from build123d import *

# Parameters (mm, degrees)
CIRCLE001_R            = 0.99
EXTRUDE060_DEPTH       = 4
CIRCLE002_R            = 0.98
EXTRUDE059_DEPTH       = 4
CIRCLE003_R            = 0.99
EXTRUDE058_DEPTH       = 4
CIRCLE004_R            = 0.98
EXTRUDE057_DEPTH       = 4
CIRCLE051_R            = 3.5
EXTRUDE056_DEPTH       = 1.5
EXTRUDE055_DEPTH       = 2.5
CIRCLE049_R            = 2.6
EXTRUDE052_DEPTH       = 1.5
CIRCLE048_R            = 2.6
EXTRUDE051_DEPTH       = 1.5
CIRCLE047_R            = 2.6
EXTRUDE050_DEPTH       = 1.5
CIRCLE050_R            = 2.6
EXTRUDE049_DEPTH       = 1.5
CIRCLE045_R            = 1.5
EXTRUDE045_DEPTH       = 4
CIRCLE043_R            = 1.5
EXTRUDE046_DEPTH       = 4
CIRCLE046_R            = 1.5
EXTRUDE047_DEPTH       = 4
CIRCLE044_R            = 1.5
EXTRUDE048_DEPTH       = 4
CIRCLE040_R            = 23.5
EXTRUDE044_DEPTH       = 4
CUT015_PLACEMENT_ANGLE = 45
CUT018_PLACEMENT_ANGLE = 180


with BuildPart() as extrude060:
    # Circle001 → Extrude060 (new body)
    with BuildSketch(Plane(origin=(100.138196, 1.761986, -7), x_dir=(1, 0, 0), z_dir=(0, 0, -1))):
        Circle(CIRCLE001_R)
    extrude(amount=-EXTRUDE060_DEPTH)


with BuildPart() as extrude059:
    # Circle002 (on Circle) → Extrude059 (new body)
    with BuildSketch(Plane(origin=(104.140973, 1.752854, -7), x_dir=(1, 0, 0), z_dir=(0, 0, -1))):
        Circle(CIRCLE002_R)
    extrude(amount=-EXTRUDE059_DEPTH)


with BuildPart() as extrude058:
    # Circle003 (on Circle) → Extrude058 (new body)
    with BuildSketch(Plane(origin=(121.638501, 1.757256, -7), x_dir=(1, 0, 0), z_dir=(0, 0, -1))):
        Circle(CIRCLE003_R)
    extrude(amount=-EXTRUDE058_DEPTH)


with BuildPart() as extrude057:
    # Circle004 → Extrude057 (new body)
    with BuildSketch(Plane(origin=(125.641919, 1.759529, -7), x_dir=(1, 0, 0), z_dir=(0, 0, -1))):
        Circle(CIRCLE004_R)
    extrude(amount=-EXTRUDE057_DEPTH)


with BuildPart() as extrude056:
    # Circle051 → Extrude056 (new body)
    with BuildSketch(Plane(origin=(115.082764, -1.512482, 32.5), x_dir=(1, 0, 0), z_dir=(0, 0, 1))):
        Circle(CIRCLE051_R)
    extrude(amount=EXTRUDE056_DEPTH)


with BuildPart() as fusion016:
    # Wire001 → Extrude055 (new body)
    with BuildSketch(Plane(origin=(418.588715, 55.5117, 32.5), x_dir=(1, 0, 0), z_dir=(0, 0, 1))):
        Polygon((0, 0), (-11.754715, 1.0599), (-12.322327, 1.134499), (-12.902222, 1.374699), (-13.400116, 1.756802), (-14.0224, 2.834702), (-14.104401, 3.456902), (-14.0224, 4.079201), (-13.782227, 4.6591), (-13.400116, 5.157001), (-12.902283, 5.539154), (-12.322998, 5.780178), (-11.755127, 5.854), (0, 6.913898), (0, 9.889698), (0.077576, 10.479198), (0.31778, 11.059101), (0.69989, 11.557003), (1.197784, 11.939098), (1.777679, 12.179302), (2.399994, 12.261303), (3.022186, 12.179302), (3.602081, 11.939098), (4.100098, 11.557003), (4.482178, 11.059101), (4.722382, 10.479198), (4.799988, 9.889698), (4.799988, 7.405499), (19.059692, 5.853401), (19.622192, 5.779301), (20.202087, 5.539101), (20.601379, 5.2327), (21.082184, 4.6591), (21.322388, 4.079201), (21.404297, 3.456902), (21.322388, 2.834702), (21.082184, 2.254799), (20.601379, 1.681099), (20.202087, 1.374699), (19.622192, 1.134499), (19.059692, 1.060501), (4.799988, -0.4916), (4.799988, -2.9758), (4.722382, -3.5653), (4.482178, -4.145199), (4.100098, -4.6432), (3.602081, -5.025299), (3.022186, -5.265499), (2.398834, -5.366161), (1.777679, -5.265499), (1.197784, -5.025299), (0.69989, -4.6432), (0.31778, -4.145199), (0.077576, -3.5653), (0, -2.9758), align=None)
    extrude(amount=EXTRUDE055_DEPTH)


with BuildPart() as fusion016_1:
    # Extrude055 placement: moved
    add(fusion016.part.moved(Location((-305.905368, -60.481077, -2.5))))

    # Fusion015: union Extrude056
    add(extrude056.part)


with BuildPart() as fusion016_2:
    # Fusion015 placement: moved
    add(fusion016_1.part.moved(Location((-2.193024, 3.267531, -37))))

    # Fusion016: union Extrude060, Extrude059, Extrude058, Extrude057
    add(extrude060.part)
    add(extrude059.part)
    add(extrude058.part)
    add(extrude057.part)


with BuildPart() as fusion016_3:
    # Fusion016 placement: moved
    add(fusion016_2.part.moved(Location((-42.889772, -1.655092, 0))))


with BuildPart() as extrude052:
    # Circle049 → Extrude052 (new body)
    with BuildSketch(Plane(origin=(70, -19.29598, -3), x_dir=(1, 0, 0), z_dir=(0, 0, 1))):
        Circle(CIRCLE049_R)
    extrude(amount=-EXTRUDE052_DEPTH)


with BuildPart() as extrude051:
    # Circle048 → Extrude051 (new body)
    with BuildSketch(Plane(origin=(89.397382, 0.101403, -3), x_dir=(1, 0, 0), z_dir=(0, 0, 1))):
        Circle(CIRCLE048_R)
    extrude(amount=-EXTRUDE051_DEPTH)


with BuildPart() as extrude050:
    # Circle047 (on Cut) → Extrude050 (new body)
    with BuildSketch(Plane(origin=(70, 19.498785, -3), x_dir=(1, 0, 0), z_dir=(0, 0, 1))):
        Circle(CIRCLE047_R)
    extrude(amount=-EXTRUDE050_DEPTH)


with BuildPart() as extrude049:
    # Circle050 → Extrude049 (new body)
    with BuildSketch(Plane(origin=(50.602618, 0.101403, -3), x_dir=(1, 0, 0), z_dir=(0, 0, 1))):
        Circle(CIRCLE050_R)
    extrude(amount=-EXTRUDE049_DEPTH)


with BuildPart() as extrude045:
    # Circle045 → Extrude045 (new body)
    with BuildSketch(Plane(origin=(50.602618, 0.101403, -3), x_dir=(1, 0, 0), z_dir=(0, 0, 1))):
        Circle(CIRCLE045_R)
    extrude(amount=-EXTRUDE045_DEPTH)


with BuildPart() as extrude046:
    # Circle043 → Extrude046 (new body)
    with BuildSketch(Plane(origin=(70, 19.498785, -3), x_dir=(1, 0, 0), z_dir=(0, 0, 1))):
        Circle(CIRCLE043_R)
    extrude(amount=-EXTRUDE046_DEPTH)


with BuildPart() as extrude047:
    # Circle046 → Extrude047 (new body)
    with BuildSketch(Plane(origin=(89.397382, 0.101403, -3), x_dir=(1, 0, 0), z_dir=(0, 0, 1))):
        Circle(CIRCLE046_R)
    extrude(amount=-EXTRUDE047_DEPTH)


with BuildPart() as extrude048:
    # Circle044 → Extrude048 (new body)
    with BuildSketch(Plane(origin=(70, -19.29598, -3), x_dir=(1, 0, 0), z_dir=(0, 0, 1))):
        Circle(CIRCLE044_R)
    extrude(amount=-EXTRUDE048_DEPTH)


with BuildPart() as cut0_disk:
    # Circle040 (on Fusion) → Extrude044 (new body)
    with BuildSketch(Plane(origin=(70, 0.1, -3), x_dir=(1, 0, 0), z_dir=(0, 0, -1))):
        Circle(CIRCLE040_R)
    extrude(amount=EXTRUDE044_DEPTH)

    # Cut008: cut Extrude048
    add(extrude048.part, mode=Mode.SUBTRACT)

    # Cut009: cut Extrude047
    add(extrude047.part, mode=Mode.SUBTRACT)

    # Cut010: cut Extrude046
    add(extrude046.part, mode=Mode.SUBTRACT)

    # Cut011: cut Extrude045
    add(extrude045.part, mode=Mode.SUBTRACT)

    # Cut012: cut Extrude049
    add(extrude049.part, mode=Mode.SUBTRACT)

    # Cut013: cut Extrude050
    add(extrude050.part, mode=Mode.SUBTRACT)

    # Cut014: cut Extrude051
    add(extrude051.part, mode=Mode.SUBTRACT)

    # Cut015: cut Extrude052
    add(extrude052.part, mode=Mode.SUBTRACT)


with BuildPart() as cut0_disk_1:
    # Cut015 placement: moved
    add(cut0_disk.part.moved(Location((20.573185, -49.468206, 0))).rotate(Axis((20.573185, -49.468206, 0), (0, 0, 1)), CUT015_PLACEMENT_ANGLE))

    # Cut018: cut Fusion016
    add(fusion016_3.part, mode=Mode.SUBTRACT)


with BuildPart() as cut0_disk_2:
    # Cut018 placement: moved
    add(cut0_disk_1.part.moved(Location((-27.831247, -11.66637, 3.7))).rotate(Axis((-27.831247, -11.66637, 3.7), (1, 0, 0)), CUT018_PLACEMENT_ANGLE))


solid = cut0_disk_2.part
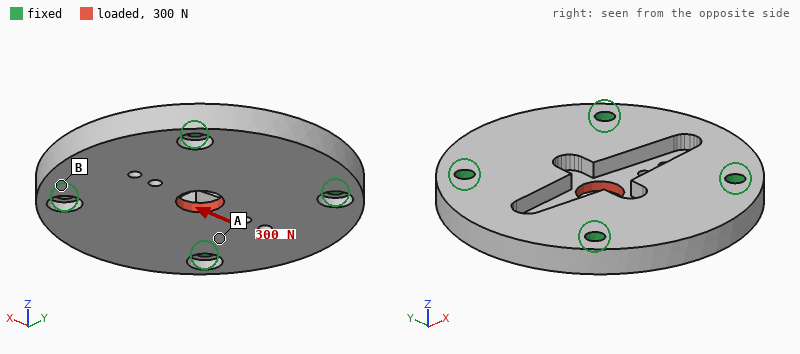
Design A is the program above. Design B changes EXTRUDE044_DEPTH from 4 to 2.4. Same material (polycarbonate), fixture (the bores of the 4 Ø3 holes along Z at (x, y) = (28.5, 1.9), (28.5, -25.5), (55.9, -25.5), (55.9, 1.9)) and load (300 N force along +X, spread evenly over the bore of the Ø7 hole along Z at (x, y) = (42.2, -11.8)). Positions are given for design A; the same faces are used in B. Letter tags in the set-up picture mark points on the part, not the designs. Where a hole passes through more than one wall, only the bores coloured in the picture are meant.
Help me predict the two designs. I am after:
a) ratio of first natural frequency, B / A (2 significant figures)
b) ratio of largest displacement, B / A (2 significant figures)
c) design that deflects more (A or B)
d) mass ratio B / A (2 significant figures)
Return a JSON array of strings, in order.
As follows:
["0.60", "1.3", "B", "0.61"]
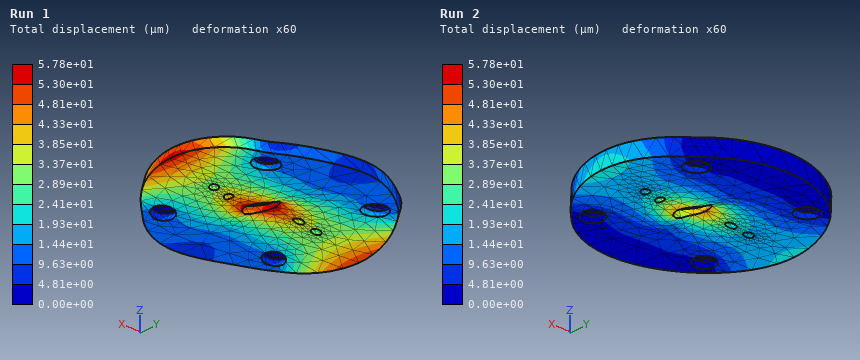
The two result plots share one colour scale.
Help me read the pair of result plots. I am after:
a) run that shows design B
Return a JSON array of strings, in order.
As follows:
["Run 1"]
